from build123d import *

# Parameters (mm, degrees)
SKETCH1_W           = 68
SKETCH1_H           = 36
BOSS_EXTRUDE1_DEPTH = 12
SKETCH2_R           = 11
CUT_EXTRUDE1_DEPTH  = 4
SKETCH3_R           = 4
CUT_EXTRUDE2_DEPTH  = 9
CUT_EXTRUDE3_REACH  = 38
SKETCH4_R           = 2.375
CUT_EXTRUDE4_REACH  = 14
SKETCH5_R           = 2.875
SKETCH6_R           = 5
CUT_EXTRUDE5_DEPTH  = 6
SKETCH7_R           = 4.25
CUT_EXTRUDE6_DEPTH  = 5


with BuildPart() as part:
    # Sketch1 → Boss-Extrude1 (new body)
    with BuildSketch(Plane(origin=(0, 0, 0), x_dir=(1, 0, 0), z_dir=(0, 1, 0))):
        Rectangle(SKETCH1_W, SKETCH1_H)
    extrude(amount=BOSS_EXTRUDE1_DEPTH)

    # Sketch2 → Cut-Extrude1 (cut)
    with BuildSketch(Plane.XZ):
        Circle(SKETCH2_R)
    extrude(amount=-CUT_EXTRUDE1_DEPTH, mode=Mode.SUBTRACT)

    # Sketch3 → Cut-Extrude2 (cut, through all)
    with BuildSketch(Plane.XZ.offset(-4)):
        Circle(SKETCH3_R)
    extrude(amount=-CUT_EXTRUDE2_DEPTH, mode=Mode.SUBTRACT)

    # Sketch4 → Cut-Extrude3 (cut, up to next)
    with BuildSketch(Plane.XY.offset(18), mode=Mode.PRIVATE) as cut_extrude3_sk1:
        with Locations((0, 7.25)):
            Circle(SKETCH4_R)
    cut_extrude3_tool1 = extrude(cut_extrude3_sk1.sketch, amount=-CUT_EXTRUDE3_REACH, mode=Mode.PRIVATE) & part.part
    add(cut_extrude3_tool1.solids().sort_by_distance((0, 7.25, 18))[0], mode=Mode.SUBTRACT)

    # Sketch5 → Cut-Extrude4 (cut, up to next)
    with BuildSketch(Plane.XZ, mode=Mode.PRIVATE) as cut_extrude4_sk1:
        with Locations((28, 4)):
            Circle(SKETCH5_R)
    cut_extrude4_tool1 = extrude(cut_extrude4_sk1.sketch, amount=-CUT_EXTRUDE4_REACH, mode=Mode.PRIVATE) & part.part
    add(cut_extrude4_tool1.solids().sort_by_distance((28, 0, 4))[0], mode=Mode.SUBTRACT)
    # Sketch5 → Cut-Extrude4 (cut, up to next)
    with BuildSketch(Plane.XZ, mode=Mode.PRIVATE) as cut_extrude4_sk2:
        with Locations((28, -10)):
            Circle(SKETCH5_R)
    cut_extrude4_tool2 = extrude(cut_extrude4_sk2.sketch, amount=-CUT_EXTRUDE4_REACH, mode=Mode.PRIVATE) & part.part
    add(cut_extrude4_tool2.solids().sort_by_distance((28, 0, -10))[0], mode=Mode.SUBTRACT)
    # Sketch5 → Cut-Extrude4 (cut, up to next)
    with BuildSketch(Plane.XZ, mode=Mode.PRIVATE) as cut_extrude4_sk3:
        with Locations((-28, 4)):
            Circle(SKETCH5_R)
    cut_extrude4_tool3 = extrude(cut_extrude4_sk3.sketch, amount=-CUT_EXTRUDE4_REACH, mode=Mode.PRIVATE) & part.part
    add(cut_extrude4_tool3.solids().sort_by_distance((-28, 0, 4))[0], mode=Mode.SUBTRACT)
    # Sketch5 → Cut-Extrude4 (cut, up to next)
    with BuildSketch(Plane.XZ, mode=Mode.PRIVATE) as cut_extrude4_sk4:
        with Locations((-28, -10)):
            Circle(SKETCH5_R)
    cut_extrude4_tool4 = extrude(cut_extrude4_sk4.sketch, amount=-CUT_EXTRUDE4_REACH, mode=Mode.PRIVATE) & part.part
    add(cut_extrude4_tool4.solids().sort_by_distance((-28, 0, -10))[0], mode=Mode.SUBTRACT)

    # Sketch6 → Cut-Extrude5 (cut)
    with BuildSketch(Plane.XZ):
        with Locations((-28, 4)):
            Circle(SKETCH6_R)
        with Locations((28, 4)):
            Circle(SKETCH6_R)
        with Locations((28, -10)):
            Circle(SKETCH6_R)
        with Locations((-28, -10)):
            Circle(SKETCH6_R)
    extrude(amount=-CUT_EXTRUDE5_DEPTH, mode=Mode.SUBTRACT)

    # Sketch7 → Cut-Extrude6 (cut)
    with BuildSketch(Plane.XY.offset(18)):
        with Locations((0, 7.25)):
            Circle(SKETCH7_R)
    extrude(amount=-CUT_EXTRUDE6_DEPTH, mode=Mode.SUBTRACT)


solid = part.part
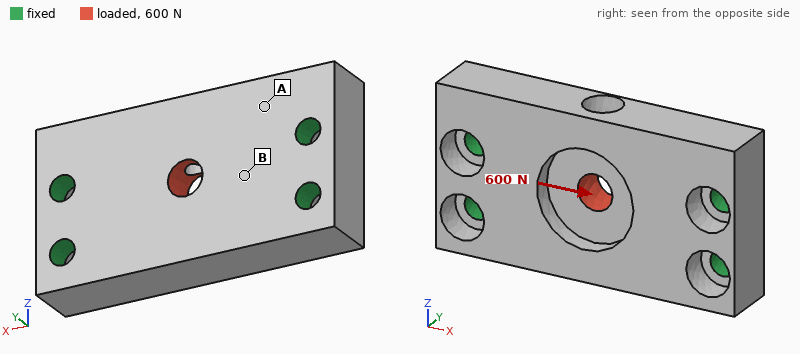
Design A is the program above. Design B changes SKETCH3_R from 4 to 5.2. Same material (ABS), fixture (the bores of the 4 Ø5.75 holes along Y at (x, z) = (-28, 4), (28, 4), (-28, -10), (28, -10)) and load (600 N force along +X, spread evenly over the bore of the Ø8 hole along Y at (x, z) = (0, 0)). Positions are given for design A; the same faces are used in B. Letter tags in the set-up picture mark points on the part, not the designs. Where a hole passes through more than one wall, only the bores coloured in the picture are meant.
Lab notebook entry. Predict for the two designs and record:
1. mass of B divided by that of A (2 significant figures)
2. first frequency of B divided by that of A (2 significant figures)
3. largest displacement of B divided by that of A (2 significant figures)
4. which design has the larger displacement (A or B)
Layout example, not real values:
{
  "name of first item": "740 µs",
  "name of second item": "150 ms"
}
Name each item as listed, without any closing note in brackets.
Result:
{
  "mass of B divided by that of A": "0.99",
  "first frequency of B divided by that of A": "1.0",
  "largest displacement of B divided by that of A": "0.89",
  "which design has the larger displacement": "A"
}
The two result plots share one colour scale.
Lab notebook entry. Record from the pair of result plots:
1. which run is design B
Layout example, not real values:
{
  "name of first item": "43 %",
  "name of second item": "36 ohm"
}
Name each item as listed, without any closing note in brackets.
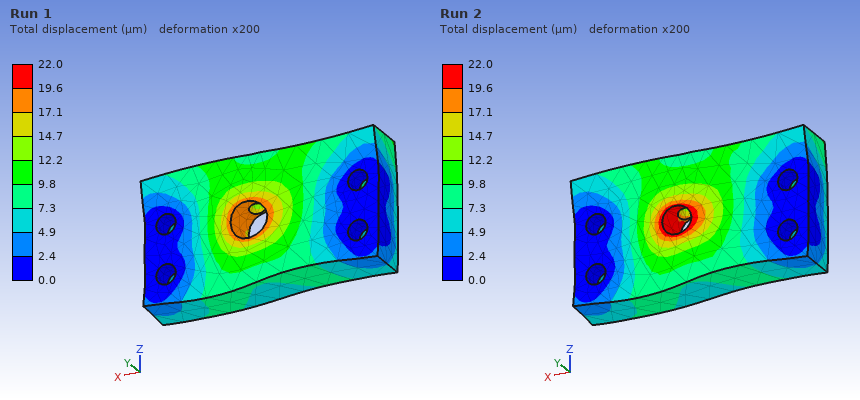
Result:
{
  "which run is design B": "Run 1"
}
